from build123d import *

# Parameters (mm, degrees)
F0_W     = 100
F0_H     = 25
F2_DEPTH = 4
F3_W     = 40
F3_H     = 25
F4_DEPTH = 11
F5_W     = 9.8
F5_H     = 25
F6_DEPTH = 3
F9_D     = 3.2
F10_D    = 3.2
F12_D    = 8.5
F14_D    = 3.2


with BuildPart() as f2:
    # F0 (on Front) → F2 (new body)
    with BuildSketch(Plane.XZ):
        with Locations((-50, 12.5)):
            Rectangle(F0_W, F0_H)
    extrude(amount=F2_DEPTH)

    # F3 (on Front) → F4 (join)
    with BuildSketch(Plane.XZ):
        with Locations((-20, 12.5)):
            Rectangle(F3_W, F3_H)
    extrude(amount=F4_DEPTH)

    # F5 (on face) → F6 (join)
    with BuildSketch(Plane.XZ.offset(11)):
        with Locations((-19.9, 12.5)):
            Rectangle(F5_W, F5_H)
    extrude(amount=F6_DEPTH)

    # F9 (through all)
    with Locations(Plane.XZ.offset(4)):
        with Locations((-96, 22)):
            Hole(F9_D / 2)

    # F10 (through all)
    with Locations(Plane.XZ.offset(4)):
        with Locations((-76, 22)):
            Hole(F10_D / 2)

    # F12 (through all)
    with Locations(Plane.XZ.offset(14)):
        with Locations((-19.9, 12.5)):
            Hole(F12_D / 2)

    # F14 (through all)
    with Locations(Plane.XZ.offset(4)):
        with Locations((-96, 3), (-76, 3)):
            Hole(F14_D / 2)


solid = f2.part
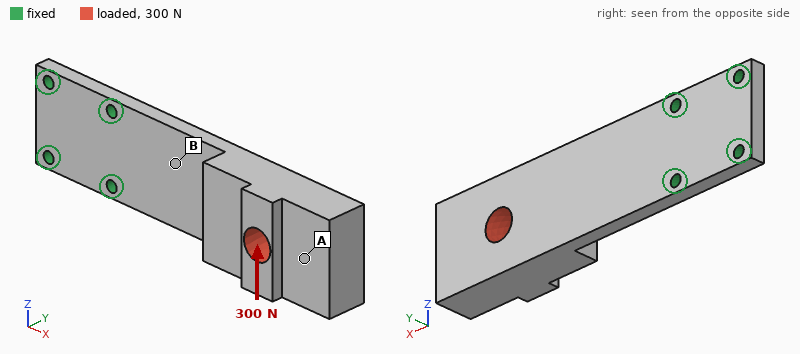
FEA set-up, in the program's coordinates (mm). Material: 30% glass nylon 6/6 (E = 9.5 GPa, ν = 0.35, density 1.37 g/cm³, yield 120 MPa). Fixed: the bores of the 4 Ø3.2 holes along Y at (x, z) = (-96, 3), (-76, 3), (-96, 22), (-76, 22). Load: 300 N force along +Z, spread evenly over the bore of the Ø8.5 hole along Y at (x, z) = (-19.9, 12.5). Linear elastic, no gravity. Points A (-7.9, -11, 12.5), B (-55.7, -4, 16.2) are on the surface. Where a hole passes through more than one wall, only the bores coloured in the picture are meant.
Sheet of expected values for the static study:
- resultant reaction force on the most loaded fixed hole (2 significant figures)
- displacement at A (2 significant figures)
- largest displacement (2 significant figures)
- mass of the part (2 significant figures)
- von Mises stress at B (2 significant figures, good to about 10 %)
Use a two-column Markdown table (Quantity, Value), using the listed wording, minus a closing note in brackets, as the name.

| Quantity | Value |
|---|---|
| resultant reaction force on the most loaded fixed hole | 840 N |
| displacement at A | 0.69 mm |
| largest displacement | 0.81 mm |
| mass of the part | 23 g |
| von Mises stress at B | 27 MPa |
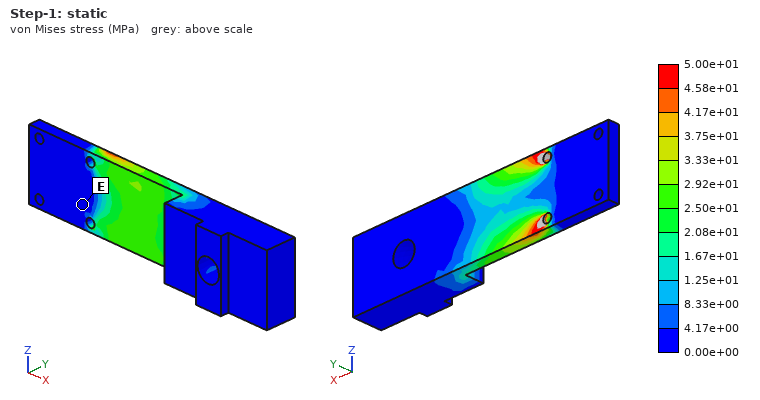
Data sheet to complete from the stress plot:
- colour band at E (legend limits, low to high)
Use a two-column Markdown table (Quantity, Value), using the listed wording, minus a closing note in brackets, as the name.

| Quantity | Value |
|---|---|
| colour band at E | 0.00e+00 to 4.17e+00 MPa |
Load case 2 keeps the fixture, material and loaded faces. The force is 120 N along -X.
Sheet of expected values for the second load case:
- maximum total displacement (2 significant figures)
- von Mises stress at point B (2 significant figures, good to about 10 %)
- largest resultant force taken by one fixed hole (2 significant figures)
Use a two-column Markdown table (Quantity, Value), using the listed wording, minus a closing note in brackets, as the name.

| Quantity | Value |
|---|---|
| maximum total displacement | 1.0 mm |
| von Mises stress at point B | 9.8 MPa |
| largest resultant force taken by one fixed hole | 54 N |
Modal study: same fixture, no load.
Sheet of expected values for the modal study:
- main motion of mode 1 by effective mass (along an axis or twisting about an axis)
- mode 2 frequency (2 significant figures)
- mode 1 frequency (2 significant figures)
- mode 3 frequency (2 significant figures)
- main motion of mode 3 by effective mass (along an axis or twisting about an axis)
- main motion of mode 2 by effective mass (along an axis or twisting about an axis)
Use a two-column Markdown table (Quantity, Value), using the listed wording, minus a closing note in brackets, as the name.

| Quantity | Value |
|---|---|
| main motion of mode 1 by effective mass | along Y |
| mode 2 frequency | 940 Hz |
| mode 1 frequency | 190 Hz |
| mode 3 frequency | 1400 Hz |
| main motion of mode 3 by effective mass | along Z |
| main motion of mode 2 by effective mass | along Z |
